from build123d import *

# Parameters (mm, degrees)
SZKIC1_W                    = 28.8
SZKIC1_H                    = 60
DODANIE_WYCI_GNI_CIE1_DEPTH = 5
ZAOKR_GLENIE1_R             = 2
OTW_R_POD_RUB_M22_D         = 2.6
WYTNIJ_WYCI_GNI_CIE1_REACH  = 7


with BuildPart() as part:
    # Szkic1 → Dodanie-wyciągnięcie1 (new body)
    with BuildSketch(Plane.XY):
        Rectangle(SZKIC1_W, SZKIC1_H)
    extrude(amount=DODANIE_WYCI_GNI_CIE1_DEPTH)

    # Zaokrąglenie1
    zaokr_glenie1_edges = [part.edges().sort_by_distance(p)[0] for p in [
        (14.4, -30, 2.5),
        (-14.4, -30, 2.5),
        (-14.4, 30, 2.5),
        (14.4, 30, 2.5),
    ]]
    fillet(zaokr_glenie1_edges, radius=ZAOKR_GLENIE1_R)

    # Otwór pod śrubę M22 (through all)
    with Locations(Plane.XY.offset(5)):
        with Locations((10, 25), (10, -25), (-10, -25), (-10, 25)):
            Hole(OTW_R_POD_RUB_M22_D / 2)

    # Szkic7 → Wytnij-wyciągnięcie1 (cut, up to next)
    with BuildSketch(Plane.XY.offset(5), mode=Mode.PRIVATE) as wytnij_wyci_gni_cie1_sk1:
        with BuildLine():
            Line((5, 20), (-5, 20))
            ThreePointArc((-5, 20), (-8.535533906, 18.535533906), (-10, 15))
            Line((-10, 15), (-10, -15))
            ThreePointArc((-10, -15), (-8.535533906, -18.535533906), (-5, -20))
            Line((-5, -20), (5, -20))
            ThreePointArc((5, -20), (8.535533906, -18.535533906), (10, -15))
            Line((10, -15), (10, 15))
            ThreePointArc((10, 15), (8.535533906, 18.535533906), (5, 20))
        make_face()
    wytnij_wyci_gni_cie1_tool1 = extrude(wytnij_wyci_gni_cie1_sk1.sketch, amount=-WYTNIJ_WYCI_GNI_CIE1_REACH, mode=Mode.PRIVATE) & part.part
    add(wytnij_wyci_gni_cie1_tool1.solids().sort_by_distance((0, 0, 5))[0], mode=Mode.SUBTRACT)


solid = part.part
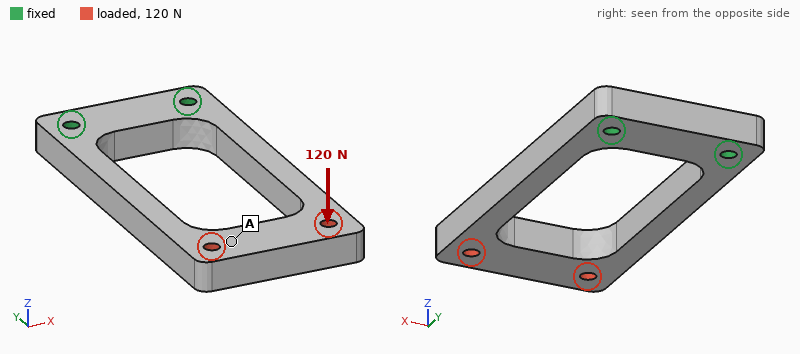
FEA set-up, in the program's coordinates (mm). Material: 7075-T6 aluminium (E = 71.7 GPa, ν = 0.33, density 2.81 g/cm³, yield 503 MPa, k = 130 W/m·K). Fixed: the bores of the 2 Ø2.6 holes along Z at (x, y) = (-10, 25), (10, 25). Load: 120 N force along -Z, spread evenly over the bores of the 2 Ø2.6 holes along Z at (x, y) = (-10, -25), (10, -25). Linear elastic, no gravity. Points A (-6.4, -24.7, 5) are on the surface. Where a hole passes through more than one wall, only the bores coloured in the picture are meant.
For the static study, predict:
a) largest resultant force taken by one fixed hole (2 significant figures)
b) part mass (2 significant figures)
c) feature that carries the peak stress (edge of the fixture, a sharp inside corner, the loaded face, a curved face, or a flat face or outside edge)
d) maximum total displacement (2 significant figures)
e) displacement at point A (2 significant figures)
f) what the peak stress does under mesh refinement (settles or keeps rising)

60 N
13 g
edge of the fixture
0.76 mm
0.65 mm
keeps rising
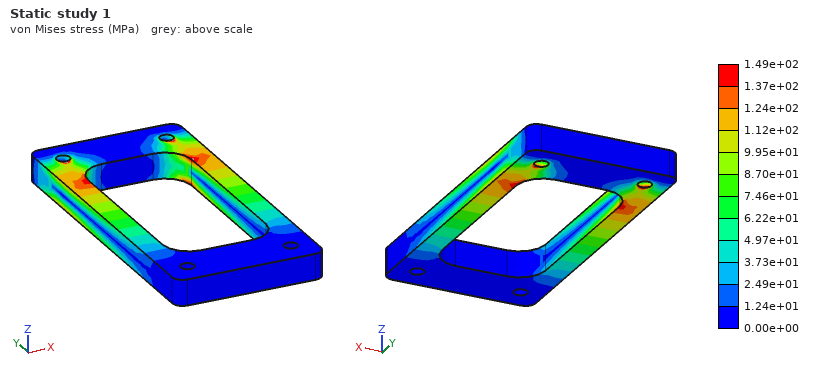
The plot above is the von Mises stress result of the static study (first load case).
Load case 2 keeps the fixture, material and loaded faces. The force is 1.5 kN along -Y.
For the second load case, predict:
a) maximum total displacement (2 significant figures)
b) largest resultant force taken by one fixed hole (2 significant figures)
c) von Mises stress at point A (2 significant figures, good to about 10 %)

28 µm
750 N
8.2 MPa
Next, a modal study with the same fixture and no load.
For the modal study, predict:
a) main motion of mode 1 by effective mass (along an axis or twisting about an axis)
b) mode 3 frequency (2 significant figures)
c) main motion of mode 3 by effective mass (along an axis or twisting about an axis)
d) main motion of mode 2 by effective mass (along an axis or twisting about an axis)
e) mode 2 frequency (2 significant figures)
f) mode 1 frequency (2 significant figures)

along Z
3000 Hz
twisting about Y
along X
1900 Hz
970 Hz
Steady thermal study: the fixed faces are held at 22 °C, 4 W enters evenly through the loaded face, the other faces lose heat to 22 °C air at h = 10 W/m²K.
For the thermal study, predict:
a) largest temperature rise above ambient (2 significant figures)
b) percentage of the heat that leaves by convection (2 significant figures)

29 K
11 %
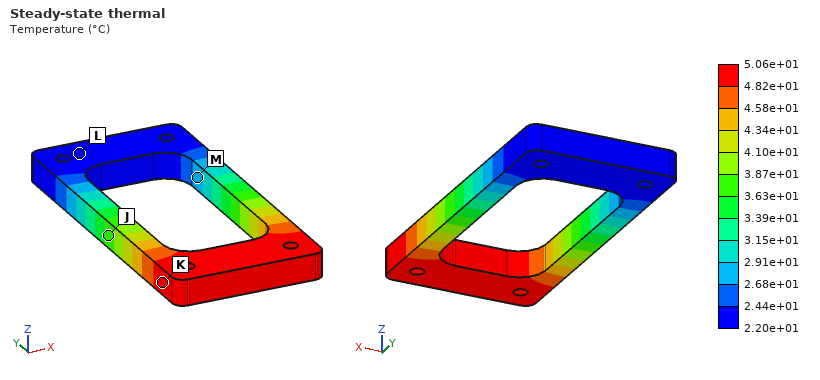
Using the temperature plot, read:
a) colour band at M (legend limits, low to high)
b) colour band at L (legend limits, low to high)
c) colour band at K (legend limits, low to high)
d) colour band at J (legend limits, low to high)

2.68e+01 to 2.91e+01 °C
2.20e+01 to 2.44e+01 °C
4.82e+01 to 5.06e+01 °C
3.63e+01 to 3.87e+01 °C
